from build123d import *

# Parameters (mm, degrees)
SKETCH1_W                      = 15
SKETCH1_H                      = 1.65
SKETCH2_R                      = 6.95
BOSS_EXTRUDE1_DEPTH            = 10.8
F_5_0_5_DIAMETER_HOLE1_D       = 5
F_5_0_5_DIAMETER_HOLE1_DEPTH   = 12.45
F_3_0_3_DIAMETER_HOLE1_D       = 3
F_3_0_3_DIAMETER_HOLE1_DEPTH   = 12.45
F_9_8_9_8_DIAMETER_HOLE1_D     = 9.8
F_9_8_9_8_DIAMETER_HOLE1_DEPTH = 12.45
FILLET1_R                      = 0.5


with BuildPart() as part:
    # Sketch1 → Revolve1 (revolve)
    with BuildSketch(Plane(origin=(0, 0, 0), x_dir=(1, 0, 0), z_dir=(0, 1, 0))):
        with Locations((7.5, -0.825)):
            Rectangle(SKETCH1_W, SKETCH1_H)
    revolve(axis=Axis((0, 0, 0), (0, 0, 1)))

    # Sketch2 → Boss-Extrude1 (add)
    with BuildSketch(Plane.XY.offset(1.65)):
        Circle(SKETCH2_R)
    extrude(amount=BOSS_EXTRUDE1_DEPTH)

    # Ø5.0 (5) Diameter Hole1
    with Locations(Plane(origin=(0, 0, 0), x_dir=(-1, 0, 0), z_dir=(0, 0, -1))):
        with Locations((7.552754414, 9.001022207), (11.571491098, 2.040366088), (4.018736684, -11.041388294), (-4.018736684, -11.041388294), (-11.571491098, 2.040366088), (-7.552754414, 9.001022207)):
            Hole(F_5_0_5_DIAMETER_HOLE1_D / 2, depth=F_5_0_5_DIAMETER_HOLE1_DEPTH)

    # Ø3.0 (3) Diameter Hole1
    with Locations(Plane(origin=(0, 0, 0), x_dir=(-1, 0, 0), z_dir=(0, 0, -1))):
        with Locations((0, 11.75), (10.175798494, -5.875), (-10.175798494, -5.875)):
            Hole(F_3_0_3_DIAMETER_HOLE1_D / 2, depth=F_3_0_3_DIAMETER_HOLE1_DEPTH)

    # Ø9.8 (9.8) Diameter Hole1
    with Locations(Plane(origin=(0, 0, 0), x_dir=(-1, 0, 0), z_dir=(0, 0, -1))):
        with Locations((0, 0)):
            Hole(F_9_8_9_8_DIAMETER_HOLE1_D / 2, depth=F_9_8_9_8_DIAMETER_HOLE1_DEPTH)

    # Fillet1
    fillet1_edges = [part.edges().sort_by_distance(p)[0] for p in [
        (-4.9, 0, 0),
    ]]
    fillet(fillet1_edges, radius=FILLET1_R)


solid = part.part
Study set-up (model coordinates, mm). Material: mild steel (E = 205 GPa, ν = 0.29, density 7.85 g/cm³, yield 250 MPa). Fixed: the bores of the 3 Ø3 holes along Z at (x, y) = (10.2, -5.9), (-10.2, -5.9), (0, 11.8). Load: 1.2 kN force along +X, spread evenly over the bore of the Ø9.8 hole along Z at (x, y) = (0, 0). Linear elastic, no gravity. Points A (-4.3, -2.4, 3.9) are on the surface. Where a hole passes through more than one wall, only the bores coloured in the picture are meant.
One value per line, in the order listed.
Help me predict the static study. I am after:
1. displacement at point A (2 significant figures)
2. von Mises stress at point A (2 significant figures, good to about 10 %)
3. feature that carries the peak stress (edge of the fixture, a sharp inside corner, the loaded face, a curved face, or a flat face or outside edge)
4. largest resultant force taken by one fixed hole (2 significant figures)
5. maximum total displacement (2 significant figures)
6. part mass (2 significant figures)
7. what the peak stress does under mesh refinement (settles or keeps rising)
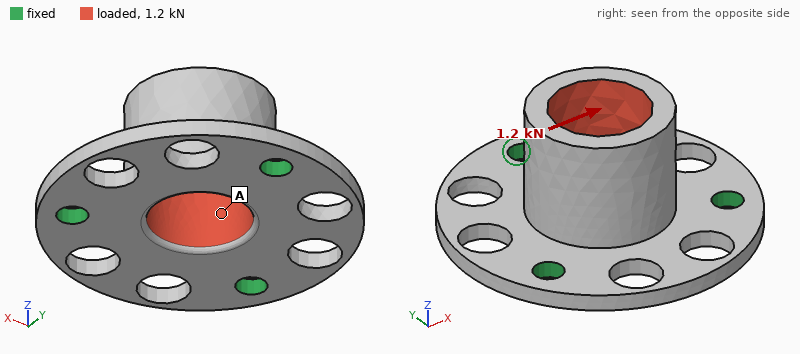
6.3 µm
32 MPa
edge of the fixture
600 N
19 µm
13 g
keeps rising
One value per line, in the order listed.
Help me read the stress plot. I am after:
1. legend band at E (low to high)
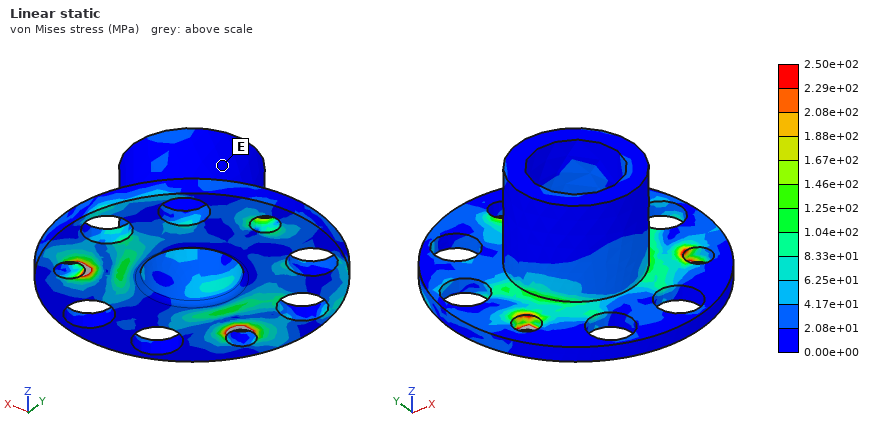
0.00e+00 to 2.08e+01 MPa
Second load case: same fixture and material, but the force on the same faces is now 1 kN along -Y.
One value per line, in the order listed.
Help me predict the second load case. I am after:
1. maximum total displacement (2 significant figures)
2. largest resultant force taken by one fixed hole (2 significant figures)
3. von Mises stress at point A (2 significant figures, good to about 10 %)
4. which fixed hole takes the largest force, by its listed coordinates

17 µm
560 N
27 MPa
(0, 11.8)
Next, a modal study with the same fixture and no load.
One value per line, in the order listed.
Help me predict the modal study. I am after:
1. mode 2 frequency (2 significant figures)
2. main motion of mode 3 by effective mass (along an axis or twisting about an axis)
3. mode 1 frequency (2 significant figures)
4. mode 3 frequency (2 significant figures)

15 kHz
along Z
15 kHz
18 kHz
